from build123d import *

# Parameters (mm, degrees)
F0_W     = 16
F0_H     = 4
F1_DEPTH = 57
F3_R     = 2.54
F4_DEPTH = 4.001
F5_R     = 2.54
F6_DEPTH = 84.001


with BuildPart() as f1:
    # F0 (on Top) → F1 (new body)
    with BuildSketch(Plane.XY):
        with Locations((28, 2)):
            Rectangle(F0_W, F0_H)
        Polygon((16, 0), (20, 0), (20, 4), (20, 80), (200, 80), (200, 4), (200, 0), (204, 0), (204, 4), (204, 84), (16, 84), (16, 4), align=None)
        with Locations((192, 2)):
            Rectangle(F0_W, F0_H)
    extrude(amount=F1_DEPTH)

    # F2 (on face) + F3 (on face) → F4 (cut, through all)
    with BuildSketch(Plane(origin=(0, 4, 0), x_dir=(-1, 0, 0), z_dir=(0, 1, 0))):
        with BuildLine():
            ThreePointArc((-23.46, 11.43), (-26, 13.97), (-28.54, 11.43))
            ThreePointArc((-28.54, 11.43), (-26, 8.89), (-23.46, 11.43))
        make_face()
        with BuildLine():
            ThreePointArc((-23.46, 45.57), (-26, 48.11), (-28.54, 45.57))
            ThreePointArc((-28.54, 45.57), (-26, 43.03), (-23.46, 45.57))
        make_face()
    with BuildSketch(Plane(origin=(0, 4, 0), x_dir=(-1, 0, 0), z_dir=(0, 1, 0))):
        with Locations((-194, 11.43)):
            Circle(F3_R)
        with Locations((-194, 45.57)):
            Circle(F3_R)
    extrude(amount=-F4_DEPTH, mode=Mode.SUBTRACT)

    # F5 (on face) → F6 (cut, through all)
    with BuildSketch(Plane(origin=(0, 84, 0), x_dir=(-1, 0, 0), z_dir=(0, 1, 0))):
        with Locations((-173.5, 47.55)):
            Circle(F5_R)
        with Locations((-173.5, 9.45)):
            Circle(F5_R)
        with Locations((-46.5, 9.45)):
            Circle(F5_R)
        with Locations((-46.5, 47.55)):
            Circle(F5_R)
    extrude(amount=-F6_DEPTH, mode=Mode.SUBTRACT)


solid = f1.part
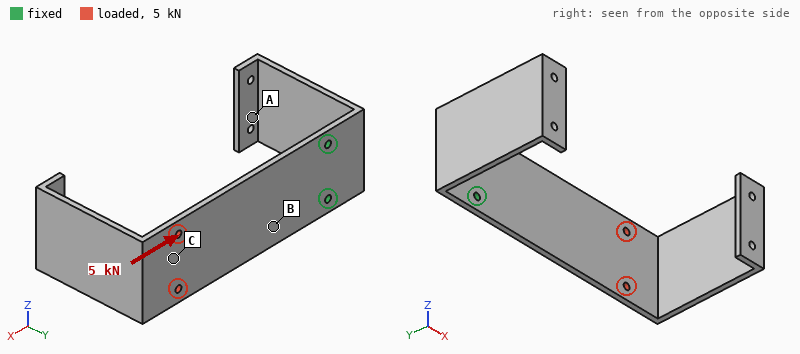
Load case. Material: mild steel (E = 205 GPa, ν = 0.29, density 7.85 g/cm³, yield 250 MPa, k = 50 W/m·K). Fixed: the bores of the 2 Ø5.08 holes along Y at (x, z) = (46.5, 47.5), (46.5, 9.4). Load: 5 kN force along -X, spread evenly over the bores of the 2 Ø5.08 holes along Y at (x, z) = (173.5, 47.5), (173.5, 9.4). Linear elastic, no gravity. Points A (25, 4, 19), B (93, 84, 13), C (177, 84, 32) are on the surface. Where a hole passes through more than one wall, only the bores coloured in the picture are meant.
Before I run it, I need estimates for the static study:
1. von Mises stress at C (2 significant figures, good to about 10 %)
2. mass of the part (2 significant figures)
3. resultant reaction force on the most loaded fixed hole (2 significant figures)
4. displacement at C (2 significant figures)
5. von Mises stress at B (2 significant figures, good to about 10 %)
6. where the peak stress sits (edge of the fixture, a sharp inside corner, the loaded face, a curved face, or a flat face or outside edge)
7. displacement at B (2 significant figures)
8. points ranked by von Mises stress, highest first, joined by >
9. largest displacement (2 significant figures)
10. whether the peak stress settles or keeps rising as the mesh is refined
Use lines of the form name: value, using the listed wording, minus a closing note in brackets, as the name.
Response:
von Mises stress at C: 10 MPa
mass of the part: 680 g
resultant reaction force on the most loaded fixed hole: 2.5 kN
displacement at C: 14 µm
von Mises stress at B: 22 MPa
where the peak stress sits: edge of the fixture
displacement at B: 5.7 µm
points ranked by von Mises stress, highest first, joined by >: B > C > A
largest displacement: 16 µm
whether the peak stress settles or keeps rising as the mesh is refined: keeps rising
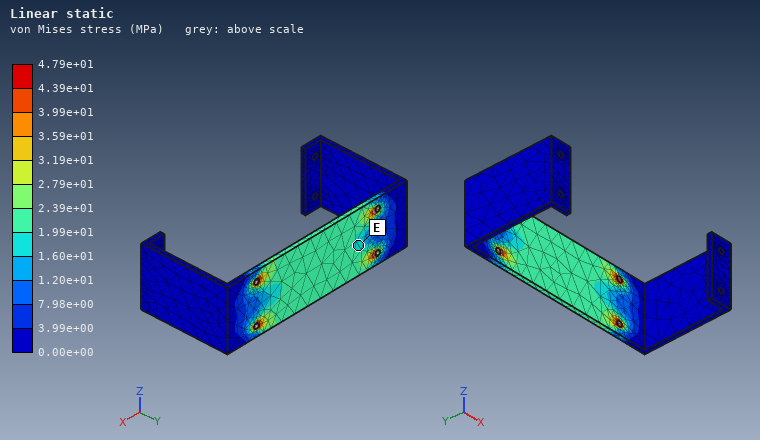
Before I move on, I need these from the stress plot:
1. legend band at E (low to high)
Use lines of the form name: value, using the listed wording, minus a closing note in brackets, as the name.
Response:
legend band at E: 1.60e+01 to 1.99e+01 MPa
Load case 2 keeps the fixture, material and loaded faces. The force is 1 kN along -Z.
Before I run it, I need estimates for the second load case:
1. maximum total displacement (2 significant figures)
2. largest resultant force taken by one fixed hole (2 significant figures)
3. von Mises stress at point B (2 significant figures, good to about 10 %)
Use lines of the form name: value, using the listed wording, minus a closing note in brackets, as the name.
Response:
maximum total displacement: 89 µm
largest resultant force taken by one fixed hole: 3.2 kN
von Mises stress at point B: 22 MPa
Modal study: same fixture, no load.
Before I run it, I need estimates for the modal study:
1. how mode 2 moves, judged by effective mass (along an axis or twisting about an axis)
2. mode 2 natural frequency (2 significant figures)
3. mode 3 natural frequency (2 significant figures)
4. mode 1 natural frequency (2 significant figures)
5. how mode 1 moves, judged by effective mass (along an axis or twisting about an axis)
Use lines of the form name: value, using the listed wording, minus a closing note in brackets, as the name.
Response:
how mode 2 moves, judged by effective mass: along Z
mode 2 natural frequency: 170 Hz
mode 3 natural frequency: 230 Hz
mode 1 natural frequency: 67 Hz
how mode 1 moves, judged by effective mass: along Y
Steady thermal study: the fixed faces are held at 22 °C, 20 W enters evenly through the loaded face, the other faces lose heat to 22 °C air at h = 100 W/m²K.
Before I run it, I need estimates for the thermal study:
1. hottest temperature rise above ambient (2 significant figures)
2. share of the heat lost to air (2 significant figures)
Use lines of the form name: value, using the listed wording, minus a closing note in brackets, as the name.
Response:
hottest temperature rise above ambient: 34 K
share of the heat lost to air: 99 %
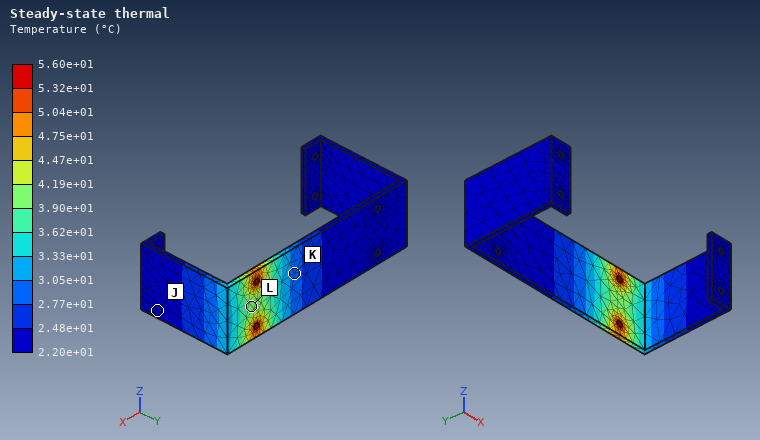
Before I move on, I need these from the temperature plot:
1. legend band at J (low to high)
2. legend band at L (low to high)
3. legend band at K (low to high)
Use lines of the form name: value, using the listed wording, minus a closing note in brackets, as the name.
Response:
legend band at J: 2.20e+01 to 2.48e+01 °C
legend band at L: 3.90e+01 to 4.19e+01 °C
legend band at K: 2.77e+01 to 3.05e+01 °C
